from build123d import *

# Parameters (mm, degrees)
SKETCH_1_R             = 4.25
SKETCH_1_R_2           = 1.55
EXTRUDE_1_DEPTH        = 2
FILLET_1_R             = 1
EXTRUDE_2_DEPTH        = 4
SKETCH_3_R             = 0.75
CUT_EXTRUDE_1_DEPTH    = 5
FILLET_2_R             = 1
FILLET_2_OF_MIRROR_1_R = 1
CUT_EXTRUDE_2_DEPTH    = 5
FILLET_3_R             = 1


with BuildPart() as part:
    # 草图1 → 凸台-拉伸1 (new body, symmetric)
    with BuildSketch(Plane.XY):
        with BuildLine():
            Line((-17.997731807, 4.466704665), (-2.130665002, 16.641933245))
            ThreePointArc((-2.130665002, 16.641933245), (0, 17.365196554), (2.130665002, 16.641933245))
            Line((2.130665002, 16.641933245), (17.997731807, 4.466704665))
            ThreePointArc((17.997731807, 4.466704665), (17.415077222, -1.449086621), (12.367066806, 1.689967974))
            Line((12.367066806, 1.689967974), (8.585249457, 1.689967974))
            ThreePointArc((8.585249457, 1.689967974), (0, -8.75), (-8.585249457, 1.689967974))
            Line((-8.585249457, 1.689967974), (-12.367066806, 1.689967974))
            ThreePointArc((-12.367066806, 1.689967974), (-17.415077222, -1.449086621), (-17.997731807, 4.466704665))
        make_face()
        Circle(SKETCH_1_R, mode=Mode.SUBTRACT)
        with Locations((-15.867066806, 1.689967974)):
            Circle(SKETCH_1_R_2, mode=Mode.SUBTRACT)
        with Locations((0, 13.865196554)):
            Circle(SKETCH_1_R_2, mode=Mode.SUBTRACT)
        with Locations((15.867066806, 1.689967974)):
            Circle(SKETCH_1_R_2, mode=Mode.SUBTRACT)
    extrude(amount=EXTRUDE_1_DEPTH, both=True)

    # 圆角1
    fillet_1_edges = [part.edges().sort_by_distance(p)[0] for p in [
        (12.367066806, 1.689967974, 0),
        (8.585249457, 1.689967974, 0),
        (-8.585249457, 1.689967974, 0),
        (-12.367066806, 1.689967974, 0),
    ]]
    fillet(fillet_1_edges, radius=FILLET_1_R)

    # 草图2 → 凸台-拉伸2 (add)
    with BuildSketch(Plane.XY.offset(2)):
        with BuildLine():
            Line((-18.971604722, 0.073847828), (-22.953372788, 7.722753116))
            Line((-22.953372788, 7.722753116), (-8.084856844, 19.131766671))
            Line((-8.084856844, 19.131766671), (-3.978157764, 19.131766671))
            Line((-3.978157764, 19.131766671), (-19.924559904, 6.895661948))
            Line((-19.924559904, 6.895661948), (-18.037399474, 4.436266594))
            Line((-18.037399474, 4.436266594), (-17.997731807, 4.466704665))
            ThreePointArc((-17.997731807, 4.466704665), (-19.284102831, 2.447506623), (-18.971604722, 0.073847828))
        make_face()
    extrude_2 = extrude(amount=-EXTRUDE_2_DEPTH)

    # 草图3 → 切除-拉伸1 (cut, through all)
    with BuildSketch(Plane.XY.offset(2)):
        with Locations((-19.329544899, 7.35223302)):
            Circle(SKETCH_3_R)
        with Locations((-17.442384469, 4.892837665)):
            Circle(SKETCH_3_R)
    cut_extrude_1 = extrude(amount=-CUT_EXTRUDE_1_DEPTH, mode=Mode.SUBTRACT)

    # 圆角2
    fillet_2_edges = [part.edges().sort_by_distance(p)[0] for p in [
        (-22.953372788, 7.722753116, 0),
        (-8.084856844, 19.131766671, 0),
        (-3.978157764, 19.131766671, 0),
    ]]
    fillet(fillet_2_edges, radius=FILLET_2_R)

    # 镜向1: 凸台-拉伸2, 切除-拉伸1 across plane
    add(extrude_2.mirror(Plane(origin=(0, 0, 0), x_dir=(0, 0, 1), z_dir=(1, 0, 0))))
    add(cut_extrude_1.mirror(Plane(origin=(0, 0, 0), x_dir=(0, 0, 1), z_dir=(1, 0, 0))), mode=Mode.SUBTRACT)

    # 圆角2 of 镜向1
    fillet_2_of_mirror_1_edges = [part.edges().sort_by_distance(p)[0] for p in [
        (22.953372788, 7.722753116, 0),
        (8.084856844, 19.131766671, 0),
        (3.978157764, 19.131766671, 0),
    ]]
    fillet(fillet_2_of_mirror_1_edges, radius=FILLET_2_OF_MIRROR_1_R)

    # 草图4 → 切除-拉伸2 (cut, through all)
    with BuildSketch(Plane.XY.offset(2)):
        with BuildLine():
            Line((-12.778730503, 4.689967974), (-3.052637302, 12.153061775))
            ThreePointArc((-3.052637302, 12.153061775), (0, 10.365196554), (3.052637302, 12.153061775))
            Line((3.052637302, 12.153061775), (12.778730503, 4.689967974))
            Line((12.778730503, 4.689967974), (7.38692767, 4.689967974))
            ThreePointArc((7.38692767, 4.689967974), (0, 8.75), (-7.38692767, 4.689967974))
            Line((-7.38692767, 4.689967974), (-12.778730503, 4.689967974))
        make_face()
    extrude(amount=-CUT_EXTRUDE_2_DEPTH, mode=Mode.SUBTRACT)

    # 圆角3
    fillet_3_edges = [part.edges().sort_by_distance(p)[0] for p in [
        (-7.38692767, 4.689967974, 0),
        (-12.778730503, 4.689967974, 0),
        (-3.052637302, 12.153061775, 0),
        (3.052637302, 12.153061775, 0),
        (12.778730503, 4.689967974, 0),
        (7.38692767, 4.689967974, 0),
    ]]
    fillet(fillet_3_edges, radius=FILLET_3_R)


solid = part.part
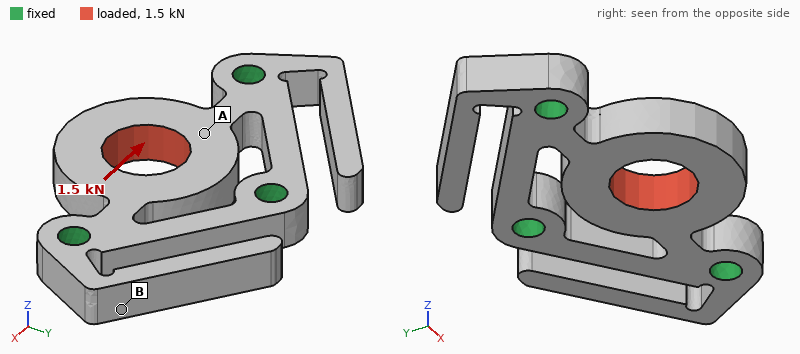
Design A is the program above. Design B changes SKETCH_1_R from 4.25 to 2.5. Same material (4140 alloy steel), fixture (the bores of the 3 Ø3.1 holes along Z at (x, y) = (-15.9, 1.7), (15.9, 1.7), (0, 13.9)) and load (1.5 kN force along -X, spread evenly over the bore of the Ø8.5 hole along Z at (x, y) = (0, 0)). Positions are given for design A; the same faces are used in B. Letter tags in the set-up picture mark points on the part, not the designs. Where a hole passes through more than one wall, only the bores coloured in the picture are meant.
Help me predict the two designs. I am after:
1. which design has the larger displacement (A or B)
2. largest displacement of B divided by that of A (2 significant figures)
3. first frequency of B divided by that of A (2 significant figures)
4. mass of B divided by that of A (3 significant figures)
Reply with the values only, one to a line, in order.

A
0.82
1.0
1.07
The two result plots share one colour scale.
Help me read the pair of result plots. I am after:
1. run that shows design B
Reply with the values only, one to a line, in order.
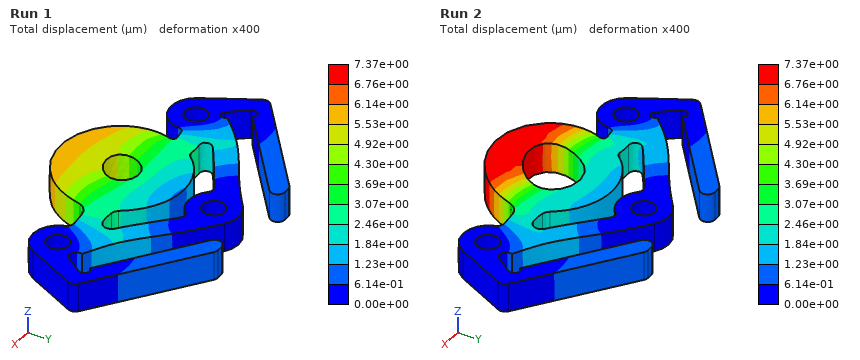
Run 1
